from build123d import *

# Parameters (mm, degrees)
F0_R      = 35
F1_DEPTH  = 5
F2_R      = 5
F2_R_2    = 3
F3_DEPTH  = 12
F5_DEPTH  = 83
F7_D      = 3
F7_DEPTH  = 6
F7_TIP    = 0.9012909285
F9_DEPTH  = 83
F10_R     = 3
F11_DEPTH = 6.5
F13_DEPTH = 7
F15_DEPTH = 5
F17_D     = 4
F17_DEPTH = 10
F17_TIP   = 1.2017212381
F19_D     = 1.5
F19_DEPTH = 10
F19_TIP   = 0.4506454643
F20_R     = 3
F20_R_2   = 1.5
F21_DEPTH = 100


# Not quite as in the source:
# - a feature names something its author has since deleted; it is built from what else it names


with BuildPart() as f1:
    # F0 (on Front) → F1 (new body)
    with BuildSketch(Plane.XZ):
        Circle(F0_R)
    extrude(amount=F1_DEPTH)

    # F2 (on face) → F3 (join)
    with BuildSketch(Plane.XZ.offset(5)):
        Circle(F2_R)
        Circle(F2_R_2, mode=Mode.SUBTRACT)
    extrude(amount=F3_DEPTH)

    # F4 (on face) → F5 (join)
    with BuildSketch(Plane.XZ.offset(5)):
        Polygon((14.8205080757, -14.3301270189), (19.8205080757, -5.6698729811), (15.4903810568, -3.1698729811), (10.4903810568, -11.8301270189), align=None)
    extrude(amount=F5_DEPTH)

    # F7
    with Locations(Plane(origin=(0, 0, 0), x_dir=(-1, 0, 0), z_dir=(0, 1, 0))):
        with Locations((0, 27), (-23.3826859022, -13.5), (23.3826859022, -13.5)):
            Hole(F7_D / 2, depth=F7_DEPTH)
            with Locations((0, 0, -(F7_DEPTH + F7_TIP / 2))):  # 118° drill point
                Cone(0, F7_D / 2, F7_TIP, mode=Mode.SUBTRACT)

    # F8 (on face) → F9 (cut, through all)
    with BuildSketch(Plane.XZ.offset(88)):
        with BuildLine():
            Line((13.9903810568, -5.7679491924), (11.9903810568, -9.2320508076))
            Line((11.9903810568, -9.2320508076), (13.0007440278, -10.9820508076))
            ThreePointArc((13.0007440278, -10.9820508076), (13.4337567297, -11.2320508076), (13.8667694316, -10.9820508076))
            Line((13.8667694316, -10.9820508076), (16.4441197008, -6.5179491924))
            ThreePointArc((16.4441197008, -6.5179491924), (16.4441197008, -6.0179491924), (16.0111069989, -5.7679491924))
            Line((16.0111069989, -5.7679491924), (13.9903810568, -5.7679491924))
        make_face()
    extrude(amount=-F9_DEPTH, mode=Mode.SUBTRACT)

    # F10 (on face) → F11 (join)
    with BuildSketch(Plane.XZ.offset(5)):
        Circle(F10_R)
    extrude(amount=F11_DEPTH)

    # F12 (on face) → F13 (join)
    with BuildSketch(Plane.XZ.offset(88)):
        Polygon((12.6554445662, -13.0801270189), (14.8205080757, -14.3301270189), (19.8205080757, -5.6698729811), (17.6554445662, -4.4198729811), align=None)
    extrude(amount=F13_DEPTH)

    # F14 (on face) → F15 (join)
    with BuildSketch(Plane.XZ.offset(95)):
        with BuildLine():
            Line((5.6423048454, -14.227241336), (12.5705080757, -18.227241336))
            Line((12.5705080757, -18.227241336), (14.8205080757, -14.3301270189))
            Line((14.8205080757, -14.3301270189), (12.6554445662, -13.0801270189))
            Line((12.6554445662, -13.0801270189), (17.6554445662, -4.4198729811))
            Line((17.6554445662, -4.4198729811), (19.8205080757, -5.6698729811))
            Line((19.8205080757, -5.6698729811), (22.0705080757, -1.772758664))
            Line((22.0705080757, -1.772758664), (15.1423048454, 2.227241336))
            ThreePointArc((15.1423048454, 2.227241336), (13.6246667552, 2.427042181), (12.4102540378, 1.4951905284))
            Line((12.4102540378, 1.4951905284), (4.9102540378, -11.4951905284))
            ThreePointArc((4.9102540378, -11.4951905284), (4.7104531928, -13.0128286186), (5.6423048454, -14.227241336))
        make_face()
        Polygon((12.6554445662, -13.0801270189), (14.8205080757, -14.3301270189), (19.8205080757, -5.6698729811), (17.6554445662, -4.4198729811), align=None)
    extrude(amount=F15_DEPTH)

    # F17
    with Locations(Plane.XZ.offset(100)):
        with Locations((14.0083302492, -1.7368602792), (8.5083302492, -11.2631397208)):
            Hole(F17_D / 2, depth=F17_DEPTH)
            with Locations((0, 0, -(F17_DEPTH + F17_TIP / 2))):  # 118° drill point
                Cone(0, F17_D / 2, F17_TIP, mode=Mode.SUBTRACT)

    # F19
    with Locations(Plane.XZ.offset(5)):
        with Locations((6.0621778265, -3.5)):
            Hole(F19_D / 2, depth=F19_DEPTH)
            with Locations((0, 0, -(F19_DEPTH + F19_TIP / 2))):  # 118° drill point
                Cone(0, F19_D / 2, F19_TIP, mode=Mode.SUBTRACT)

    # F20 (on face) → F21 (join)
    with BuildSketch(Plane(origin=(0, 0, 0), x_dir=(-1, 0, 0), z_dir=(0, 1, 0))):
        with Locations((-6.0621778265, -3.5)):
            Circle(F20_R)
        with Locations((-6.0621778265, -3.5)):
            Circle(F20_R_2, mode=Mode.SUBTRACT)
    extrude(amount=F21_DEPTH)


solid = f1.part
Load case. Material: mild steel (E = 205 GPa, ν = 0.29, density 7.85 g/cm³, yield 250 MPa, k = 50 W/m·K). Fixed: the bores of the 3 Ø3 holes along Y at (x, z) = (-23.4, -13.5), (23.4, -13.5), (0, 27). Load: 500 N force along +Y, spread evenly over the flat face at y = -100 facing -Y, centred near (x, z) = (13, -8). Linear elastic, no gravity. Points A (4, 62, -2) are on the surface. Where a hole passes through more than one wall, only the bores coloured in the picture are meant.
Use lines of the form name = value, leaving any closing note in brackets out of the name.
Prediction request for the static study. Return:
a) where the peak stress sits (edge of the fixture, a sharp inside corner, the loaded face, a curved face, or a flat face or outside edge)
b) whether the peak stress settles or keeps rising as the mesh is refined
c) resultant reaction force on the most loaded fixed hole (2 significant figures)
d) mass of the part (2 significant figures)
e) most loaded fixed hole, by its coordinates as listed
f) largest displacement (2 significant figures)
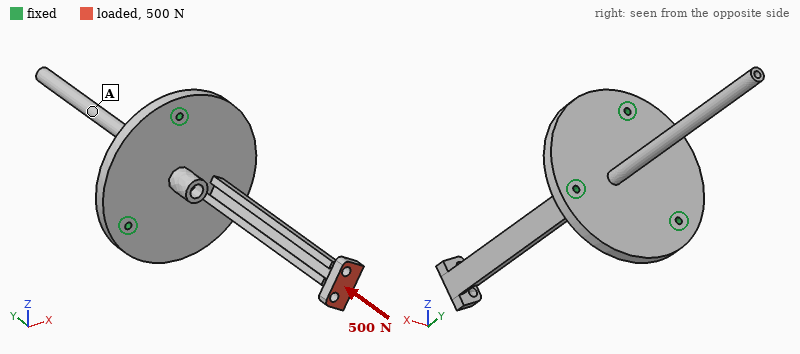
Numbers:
where the peak stress sits = a sharp inside corner
whether the peak stress settles or keeps rising as the mesh is refined = keeps rising
resultant reaction force on the most loaded fixed hole = 380 N
mass of the part = 200 g
most loaded fixed hole, by its coordinates as listed = (23.4, -13.5)
largest displacement = 0.48 mm
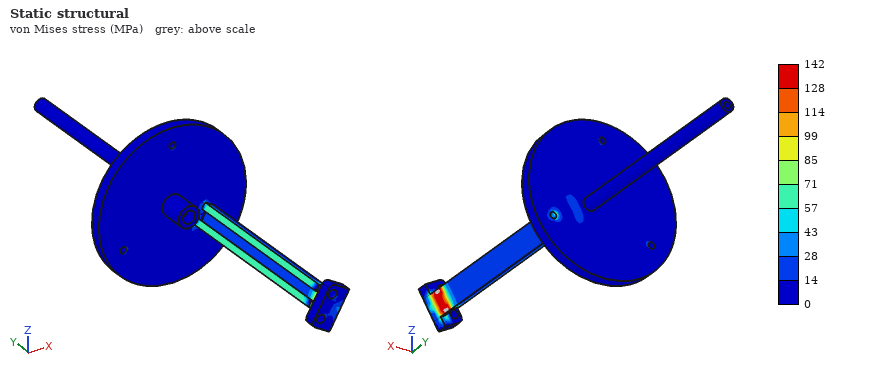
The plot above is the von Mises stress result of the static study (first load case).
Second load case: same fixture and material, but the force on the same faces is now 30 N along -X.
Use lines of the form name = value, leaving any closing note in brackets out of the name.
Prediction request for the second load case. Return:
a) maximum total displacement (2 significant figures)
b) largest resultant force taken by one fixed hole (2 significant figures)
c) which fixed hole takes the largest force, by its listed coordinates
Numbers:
maximum total displacement = 0.55 mm
largest resultant force taken by one fixed hole = 70 N
which fixed hole takes the largest force, by its listed coordinates = (23.4, -13.5)
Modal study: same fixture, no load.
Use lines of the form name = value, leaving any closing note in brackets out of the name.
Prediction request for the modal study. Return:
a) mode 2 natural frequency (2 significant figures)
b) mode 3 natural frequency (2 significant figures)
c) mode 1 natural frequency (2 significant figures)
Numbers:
mode 2 natural frequency = 460 Hz
mode 3 natural frequency = 460 Hz
mode 1 natural frequency = 340 Hz
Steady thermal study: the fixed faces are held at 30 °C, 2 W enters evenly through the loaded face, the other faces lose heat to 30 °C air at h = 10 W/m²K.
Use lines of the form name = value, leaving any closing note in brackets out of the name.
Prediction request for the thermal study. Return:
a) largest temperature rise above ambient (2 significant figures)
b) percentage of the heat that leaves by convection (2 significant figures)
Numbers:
largest temperature rise above ambient = 64 K
percentage of the heat that leaves by convection = 60 %
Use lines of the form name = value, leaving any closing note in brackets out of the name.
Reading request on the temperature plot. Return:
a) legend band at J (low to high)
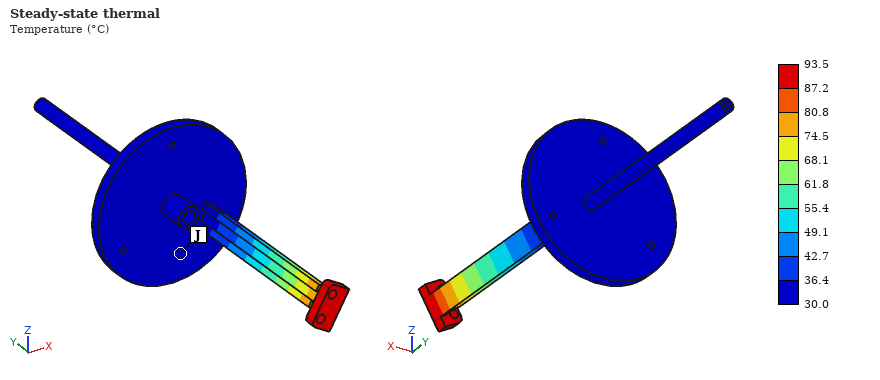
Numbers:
legend band at J = 30.0 to 36.4 °C
